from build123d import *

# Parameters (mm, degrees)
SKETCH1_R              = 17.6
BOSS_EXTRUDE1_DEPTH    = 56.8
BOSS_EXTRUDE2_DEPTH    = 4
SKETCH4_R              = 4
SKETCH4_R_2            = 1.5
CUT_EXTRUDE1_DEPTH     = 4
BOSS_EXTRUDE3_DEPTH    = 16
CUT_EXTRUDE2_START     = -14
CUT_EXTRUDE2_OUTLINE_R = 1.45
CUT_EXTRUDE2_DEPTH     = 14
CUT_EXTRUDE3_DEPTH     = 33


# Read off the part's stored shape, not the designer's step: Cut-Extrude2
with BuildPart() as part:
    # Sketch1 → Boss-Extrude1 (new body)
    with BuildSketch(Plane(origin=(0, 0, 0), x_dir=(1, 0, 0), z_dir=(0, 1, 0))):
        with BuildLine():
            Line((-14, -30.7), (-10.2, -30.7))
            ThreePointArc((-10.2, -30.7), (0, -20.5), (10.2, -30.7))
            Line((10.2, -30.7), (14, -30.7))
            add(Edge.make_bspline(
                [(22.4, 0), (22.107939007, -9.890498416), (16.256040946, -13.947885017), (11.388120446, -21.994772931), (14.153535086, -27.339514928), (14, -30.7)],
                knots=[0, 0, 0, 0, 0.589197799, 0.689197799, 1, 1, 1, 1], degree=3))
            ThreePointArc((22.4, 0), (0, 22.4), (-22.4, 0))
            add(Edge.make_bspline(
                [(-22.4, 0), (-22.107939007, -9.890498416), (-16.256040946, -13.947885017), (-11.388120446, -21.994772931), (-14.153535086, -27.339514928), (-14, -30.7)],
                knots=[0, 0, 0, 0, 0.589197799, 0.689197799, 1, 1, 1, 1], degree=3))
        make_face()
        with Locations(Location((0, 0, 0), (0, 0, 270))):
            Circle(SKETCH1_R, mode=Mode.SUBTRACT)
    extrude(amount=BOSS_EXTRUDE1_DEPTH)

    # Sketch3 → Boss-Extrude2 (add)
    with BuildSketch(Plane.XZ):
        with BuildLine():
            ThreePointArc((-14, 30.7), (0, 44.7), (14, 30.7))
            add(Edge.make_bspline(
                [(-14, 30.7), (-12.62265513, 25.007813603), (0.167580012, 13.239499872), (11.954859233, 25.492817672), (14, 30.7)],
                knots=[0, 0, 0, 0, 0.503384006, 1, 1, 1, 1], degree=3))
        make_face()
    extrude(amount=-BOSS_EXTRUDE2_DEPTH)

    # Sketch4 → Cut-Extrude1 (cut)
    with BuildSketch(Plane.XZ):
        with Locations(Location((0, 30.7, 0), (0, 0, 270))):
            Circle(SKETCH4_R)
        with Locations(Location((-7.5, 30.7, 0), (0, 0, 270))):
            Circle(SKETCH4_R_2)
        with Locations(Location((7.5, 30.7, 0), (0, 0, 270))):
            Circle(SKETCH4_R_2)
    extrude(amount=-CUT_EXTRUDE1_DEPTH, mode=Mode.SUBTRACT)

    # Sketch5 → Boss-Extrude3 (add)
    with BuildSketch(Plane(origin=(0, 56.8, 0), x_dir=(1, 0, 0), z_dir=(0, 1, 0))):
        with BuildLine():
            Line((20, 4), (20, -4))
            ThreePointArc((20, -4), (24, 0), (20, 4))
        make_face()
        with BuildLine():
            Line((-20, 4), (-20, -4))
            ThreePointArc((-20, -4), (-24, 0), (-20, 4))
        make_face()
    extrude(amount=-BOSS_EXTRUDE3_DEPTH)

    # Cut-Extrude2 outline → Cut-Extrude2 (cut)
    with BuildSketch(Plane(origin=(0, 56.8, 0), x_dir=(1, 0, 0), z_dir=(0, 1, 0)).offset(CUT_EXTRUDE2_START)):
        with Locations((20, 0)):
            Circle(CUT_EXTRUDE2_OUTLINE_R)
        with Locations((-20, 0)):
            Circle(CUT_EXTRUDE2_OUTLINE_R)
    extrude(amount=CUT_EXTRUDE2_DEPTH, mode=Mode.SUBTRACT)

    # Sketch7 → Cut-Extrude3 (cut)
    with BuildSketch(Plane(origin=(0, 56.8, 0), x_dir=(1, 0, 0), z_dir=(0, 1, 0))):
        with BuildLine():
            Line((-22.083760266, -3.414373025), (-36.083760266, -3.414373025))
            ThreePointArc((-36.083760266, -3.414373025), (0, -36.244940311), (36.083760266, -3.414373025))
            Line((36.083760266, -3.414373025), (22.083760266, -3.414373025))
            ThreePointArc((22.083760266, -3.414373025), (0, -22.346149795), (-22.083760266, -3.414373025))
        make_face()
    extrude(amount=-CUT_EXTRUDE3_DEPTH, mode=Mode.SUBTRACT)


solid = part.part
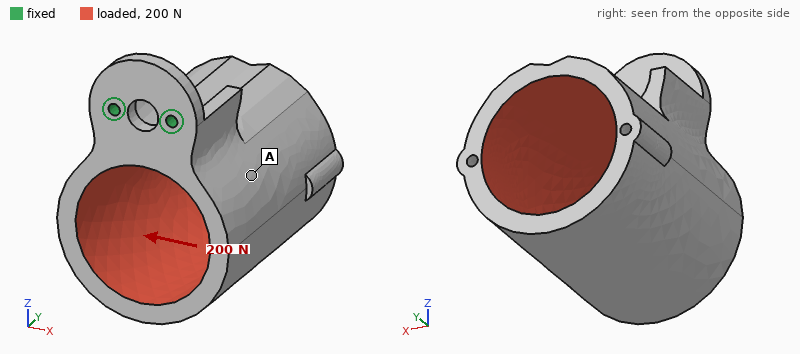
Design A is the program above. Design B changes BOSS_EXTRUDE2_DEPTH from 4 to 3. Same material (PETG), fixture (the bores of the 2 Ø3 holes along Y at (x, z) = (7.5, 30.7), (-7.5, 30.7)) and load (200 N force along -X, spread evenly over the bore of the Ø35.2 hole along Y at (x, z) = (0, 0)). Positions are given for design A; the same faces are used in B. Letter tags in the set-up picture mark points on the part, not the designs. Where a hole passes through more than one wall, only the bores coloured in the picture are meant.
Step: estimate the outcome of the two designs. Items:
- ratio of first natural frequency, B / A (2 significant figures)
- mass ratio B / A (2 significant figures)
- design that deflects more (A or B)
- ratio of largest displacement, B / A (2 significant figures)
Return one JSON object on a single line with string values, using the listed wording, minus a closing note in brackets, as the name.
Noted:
{"ratio of first natural frequency, B / A": "0.74", "mass ratio B / A": "0.99", "design that deflects more": "B", "ratio of largest displacement, B / A": "1.2"}
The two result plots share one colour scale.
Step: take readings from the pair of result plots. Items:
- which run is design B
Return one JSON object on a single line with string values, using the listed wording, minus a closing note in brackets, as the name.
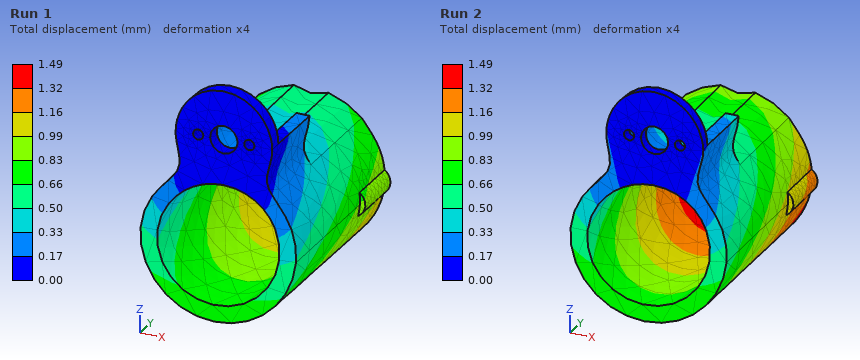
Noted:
{"which run is design B": "Run 2"}
